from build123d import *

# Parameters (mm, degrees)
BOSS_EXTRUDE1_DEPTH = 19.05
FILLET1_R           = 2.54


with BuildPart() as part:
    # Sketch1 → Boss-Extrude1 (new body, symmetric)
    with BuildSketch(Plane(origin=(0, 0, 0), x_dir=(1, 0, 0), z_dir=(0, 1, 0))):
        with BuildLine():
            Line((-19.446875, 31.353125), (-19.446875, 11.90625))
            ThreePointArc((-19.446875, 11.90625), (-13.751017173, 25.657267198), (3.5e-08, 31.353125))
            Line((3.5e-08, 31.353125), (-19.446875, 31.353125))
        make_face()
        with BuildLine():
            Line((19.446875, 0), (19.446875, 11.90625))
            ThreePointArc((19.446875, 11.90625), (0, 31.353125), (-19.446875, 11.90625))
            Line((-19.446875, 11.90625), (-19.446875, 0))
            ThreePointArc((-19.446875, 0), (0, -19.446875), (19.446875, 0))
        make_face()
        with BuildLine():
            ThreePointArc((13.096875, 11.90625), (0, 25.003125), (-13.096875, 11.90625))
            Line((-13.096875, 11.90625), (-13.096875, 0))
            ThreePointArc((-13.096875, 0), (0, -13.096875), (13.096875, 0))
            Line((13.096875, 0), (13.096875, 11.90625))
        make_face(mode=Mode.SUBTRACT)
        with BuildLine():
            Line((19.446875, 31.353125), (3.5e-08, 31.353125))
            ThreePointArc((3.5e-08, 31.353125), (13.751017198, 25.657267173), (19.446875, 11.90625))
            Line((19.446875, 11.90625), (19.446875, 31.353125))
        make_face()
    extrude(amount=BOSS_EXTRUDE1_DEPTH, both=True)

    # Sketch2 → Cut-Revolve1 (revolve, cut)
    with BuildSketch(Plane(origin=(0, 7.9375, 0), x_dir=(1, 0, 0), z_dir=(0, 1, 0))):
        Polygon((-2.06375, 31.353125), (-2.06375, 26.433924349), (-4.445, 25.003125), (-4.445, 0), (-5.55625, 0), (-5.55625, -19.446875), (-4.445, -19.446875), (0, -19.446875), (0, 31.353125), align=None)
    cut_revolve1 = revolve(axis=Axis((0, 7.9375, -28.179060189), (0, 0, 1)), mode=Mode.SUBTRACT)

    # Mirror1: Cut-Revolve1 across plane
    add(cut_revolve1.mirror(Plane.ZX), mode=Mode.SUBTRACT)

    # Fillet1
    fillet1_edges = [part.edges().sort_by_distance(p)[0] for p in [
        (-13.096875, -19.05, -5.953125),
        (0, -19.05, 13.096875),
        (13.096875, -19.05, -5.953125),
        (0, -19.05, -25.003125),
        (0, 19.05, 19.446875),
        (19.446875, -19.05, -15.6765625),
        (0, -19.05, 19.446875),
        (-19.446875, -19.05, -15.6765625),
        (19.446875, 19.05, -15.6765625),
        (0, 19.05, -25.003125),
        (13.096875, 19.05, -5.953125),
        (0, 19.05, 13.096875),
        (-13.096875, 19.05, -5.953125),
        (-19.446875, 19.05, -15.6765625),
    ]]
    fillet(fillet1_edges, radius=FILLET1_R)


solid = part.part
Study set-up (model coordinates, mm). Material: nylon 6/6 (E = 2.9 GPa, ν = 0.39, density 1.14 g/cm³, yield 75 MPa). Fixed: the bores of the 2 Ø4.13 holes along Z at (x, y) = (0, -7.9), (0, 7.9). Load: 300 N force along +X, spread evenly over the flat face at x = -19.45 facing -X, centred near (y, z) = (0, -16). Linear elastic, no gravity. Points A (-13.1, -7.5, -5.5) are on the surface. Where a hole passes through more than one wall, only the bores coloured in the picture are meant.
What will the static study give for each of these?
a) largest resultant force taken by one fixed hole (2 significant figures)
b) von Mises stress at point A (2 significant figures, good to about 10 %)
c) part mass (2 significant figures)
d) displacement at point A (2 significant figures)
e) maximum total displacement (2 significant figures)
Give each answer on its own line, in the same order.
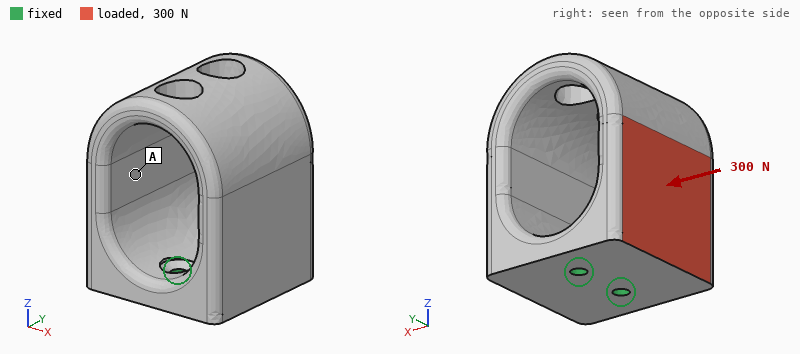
150 N
2.5 MPa
39 g
0.30 mm
0.48 mm
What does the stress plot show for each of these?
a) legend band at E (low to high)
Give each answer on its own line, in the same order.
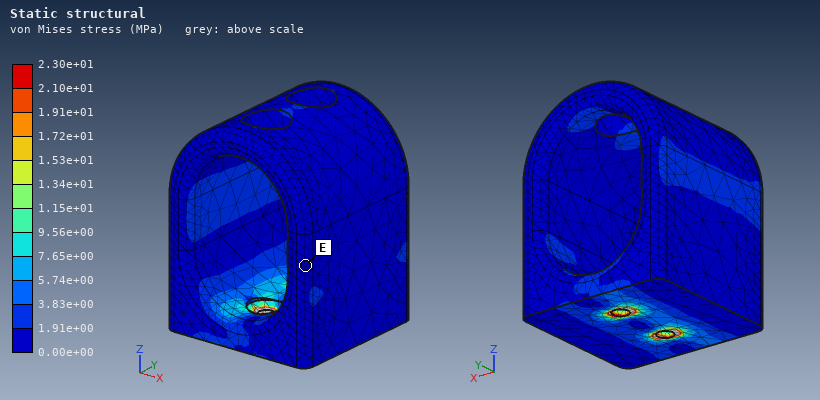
0.00e+00 to 1.91e+00 MPa
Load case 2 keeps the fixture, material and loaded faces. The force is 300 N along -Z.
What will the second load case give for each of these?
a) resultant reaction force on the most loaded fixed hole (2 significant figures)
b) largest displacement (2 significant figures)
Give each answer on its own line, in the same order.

150 N
0.62 mm
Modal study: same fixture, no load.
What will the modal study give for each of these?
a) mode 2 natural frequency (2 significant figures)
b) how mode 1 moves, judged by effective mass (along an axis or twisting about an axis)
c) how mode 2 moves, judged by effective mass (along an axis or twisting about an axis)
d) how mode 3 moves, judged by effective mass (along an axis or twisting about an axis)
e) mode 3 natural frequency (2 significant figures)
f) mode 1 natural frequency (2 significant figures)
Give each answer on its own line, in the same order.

1100 Hz
along X
along Y
along Z
1900 Hz
580 Hz
